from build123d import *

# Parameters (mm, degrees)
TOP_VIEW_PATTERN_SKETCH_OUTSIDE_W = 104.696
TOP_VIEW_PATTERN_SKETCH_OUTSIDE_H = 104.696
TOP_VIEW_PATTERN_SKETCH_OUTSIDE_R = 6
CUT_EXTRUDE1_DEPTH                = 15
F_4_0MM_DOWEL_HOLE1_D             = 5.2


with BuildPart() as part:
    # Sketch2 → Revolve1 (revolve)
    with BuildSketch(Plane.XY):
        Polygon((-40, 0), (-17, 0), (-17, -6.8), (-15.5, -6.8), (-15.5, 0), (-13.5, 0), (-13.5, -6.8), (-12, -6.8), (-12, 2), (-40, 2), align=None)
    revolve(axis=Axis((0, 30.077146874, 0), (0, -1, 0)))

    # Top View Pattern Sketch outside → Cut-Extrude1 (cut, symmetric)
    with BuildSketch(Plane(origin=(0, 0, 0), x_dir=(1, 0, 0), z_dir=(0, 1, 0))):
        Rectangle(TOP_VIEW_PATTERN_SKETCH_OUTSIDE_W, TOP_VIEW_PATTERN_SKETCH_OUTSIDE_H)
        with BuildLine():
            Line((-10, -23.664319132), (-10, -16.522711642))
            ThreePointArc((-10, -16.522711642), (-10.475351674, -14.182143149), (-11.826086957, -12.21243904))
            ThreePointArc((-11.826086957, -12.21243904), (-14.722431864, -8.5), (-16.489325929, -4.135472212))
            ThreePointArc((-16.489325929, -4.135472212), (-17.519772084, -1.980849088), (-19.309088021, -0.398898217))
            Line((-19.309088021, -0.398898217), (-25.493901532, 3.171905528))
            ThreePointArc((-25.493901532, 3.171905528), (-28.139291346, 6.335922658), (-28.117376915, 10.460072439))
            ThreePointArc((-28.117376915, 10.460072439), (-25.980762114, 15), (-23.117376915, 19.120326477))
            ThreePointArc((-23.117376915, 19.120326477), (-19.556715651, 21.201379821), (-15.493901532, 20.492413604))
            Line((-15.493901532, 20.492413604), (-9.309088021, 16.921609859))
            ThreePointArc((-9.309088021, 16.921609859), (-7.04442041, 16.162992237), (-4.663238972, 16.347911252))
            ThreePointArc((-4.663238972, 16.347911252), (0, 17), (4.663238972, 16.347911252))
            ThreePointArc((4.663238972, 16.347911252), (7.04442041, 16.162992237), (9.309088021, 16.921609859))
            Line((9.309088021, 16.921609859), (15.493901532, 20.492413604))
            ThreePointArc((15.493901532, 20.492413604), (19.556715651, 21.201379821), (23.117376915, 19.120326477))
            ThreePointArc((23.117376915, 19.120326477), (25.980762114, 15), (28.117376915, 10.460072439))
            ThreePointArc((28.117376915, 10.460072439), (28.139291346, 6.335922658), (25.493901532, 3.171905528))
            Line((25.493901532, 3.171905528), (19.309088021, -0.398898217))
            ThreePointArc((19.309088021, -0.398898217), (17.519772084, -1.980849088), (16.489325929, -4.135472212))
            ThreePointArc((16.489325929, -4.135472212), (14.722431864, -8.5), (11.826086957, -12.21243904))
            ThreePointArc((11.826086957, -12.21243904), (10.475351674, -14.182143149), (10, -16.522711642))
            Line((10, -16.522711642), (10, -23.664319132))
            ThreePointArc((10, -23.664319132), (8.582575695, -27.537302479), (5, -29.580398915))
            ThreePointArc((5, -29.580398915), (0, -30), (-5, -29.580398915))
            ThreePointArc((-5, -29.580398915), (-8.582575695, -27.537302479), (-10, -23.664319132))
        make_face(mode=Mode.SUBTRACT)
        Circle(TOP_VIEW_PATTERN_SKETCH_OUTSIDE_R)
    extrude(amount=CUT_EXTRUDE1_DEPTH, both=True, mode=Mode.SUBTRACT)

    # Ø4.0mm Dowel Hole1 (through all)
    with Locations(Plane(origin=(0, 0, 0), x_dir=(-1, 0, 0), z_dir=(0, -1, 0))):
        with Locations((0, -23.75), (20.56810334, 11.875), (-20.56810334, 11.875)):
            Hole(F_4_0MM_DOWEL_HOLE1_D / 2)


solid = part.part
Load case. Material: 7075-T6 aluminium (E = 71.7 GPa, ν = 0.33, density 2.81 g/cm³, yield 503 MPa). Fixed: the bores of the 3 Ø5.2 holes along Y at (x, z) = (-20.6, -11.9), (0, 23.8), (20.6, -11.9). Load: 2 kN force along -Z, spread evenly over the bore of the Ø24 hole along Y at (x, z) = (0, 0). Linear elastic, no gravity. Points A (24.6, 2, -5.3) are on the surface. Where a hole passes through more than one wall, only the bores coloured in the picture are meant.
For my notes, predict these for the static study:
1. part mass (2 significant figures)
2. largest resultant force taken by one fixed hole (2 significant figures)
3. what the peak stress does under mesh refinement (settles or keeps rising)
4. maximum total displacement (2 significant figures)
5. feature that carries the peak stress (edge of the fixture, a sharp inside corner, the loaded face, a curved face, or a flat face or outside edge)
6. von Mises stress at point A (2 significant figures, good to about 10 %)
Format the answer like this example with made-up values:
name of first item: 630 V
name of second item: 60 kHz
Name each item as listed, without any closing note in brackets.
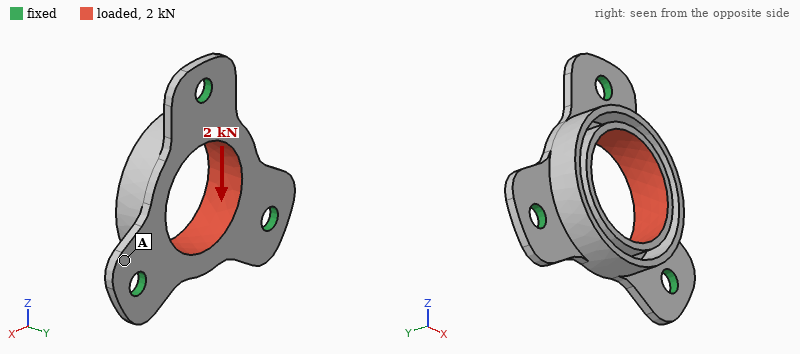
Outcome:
part mass: 12 g
largest resultant force taken by one fixed hole: 680 N
what the peak stress does under mesh refinement: keeps rising
maximum total displacement: 65 µm
feature that carries the peak stress: edge of the fixture
von Mises stress at point A: 18 MPa
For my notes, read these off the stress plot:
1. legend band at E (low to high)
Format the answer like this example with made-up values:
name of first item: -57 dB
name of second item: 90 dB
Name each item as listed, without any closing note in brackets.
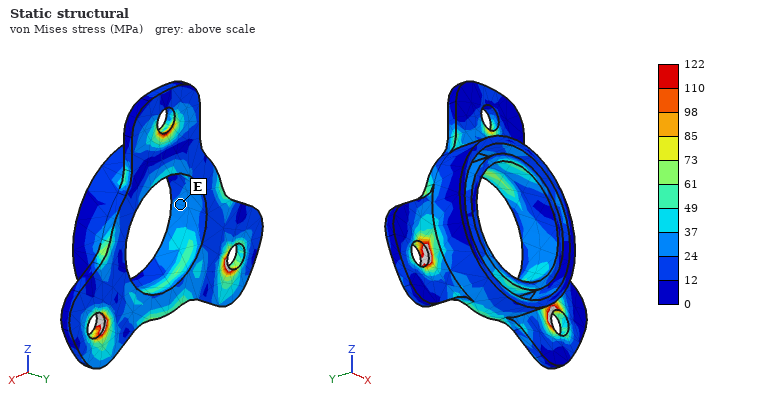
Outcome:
legend band at E: 24 to 37 MPa
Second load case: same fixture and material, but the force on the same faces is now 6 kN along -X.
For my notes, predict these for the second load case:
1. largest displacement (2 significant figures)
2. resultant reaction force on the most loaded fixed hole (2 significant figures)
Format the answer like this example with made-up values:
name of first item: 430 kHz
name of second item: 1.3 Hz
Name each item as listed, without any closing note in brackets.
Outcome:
largest displacement: 0.17 mm
resultant reaction force on the most loaded fixed hole: 2.0 kN
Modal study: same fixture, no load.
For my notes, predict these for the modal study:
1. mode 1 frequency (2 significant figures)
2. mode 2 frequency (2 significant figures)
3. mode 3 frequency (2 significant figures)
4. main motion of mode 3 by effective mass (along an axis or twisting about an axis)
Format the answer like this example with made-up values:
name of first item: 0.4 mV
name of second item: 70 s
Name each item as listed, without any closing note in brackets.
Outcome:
mode 1 frequency: 8800 Hz
mode 2 frequency: 8800 Hz
mode 3 frequency: 9500 Hz
main motion of mode 3 by effective mass: along Y
